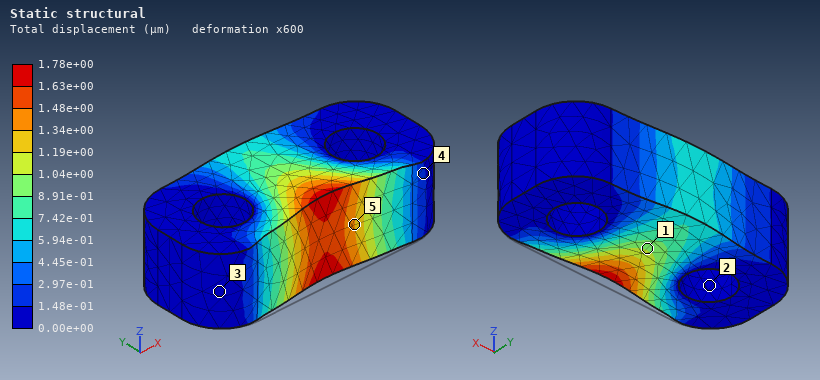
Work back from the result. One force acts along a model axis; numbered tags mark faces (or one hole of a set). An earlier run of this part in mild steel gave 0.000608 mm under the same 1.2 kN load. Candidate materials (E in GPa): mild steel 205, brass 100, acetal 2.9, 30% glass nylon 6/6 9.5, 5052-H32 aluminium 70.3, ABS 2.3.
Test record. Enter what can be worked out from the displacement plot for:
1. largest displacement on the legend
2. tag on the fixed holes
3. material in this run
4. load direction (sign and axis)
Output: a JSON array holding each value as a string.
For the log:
["1.78e+00 µm", "2", "5052-H32 aluminium", "+Y"]
